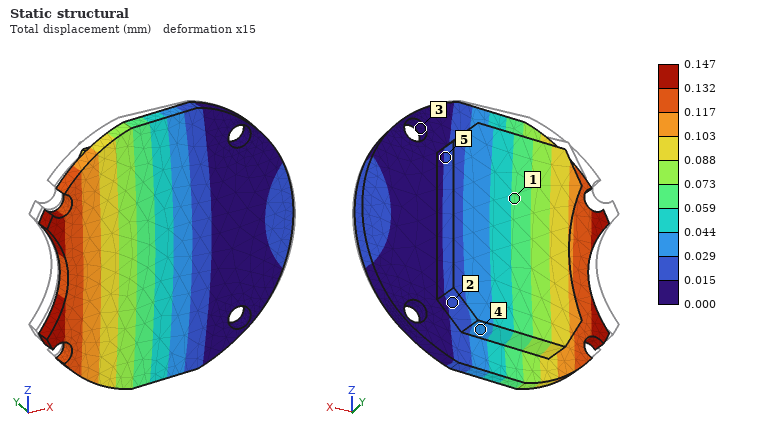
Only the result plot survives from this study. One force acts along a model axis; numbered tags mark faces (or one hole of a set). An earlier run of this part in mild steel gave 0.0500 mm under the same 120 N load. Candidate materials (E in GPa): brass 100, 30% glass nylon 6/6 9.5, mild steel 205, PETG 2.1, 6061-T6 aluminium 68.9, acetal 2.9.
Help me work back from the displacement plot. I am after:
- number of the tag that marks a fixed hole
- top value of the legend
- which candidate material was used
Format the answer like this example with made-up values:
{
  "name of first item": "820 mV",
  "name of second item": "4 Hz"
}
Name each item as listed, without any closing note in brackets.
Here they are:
{
  "number of the tag that marks a fixed hole": "3",
  "top value of the legend": "0.147 mm",
  "which candidate material was used": "6061-T6 aluminium"
}
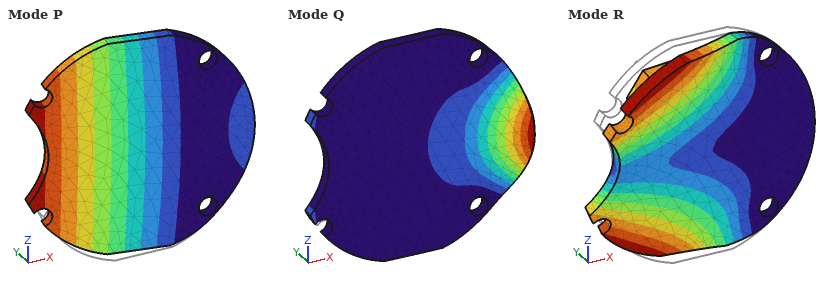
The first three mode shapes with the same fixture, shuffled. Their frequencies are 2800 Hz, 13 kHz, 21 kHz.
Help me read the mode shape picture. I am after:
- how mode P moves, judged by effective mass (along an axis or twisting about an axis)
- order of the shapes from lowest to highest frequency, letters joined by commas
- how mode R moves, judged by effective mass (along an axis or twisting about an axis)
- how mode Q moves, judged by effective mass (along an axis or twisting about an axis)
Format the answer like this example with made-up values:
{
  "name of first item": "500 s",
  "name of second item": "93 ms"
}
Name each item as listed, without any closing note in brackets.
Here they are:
{
  "how mode P moves, judged by effective mass": "along Y",
  "order of the shapes from lowest to highest frequency, letters joined by commas": "P, R, Q",
  "how mode R moves, judged by effective mass": "twisting about X",
  "how mode Q moves, judged by effective mass": "along Y"
}
